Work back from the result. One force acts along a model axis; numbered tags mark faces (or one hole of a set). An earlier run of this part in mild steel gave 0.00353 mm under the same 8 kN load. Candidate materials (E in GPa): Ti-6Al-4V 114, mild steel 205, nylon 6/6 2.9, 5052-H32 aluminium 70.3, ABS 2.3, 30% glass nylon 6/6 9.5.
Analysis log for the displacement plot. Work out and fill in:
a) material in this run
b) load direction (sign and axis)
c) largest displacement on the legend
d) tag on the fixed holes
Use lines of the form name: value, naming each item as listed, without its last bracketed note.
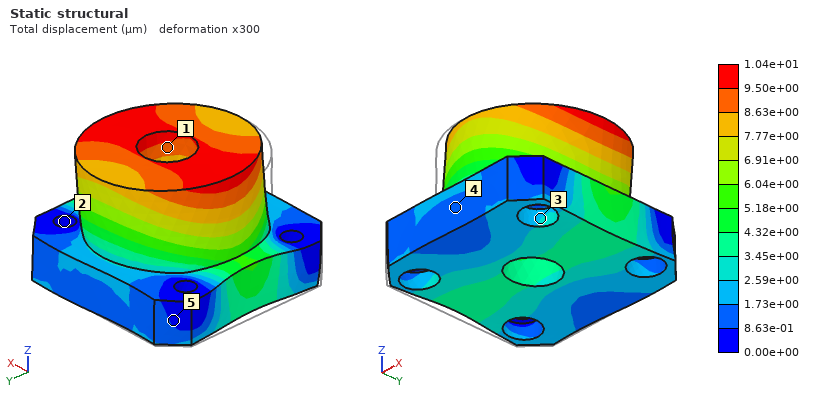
material in this run: 5052-H32 aluminium
load direction: +X
largest displacement on the legend: 1.04e+01 µm
tag on the fixed holes: 2
